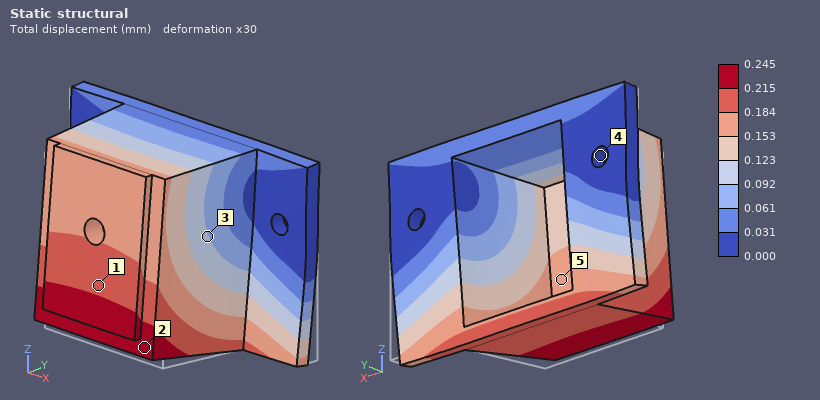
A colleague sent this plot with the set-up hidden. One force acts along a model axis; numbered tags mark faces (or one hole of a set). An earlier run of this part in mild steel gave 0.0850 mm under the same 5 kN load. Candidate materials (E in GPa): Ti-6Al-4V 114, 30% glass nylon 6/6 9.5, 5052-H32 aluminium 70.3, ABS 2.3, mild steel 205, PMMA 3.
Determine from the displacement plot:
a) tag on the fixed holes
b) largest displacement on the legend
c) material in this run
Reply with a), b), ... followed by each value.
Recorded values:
a) 4
b) 0.245 mm
c) 5052-H32 aluminium
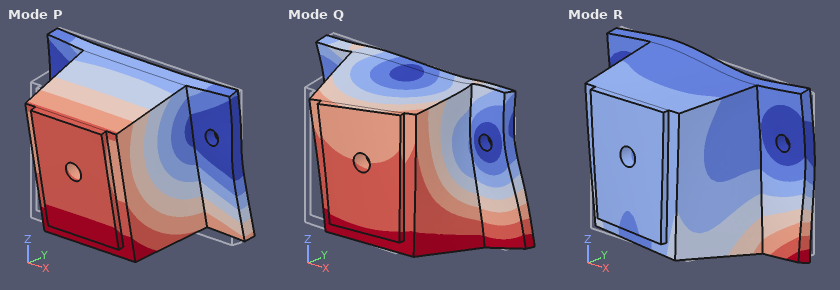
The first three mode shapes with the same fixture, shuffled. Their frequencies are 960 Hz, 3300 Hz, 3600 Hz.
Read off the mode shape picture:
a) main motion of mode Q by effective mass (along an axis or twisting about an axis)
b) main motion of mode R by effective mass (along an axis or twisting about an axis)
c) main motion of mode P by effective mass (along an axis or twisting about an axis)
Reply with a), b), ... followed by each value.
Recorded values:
a) along X
b) twisting about Z
c) along Z
